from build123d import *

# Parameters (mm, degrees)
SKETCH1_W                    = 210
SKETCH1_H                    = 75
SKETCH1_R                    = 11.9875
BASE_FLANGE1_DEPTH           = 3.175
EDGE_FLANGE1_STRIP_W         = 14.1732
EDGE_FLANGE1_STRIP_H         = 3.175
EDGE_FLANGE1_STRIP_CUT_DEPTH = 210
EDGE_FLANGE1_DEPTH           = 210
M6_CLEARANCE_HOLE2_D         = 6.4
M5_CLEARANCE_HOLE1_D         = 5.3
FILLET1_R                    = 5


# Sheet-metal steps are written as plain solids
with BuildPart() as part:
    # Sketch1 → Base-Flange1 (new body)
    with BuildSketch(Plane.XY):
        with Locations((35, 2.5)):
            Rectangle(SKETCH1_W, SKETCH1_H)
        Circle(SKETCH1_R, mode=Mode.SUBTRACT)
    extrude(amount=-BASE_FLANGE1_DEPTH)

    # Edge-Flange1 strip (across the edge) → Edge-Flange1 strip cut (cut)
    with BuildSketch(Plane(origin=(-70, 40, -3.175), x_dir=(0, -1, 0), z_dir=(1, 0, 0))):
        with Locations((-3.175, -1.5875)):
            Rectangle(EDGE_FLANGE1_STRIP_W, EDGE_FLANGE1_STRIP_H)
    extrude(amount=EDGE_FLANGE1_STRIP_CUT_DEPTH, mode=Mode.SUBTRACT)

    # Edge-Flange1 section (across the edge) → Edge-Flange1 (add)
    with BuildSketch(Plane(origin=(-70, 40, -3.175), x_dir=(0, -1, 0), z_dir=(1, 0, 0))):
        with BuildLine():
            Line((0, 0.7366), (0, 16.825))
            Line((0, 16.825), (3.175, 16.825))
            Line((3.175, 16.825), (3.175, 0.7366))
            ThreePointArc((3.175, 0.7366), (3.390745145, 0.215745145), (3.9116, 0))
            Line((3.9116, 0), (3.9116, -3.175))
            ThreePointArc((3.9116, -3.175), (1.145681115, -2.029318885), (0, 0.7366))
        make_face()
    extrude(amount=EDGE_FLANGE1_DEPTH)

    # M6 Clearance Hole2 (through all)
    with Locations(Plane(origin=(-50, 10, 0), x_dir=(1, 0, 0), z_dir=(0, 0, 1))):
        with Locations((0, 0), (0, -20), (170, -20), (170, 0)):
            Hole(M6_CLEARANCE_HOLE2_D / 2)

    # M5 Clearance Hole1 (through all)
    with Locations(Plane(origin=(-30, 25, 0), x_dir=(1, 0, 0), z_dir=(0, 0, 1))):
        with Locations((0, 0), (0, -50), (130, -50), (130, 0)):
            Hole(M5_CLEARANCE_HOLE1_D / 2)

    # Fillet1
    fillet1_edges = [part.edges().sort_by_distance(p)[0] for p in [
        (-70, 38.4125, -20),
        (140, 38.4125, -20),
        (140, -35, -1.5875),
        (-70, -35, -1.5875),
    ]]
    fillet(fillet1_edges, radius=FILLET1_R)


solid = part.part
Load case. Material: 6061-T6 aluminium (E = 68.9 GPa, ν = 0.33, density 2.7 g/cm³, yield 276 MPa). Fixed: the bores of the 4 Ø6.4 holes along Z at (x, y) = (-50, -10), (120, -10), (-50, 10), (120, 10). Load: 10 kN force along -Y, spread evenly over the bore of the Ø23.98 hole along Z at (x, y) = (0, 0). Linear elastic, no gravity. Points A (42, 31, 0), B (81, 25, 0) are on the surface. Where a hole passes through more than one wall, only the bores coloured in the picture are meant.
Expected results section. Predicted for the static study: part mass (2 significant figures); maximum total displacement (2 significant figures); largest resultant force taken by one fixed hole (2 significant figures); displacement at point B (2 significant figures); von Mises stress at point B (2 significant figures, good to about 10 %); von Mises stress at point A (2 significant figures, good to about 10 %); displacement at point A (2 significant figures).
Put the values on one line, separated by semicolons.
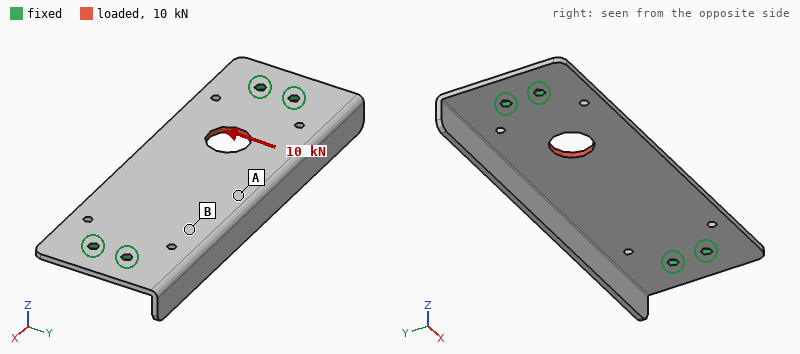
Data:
160 g; 0.24 mm; 5.1 kN; 0.085 mm; 19 MPa; 42 MPa; 0.17 mm
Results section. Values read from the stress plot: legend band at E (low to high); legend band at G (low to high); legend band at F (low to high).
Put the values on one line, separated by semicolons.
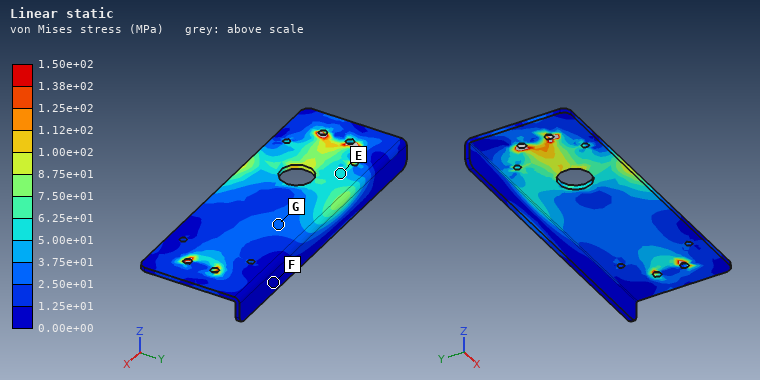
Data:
5.00e+01 to 6.25e+01 MPa; 2.50e+01 to 3.75e+01 MPa; 0.00e+00 to 1.25e+01 MPa
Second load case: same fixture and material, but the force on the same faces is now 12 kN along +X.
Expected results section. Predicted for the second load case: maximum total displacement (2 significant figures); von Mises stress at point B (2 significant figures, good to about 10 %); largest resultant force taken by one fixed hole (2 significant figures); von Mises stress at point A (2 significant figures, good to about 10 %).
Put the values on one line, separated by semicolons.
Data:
44 µm; 15 MPa; 4.0 kN; 12 MPa
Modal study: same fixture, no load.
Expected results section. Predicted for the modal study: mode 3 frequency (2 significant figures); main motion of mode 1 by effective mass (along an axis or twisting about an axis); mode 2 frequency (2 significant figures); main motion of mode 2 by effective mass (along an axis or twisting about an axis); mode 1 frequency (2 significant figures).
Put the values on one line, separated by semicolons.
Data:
1600 Hz; along Z; 980 Hz; along Z; 720 Hz
